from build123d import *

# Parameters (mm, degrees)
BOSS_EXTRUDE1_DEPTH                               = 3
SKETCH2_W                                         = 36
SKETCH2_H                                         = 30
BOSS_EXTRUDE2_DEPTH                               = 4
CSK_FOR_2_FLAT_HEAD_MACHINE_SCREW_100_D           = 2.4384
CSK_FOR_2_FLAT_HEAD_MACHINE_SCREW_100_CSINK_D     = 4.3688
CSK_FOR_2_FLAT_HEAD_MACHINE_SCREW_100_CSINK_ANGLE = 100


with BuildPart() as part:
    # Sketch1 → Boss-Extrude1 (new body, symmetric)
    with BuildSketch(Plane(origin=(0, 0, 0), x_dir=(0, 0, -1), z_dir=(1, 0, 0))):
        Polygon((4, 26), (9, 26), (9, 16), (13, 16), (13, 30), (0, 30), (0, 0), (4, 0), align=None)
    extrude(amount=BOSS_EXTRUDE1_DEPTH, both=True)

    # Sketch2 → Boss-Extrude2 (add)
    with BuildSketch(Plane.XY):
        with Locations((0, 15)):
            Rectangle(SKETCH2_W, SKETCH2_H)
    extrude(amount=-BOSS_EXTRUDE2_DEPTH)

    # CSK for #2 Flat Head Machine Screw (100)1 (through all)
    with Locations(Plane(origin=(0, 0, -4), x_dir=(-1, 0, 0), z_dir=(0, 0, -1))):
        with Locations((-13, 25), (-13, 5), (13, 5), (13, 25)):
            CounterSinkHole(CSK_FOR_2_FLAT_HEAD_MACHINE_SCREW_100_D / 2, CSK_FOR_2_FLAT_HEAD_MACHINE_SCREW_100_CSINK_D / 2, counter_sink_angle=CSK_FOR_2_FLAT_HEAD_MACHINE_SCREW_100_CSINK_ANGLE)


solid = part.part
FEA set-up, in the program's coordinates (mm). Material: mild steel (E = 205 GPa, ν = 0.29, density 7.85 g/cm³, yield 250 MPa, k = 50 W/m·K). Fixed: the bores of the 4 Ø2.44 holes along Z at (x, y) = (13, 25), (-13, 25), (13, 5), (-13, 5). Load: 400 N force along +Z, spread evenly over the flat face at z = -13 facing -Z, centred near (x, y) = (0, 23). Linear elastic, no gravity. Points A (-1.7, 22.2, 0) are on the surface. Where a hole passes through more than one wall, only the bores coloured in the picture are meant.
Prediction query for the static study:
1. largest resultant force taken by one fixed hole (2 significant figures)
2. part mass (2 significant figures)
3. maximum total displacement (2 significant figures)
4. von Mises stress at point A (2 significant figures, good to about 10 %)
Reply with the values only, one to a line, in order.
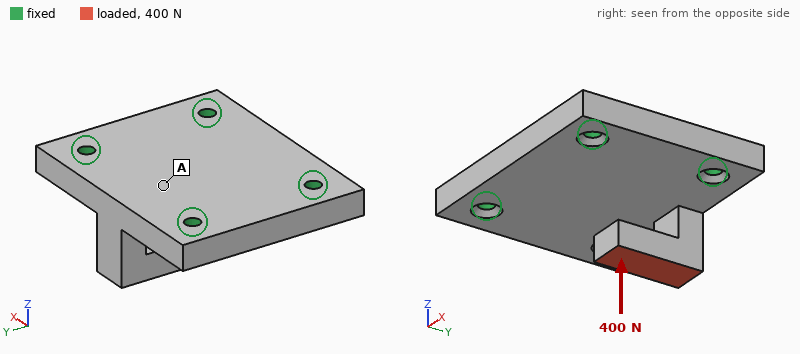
190 N
37 g
46 µm
23 MPa
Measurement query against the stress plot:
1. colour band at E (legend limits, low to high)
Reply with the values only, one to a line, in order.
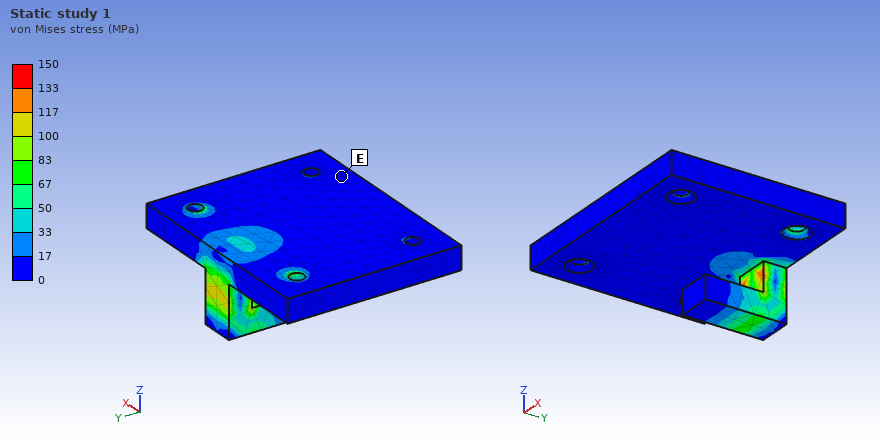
0 to 17 MPa
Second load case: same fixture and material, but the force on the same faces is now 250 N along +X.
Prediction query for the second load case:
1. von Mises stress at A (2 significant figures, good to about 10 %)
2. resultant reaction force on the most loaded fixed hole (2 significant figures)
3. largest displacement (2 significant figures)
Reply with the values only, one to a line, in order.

13 MPa
180 N
32 µm
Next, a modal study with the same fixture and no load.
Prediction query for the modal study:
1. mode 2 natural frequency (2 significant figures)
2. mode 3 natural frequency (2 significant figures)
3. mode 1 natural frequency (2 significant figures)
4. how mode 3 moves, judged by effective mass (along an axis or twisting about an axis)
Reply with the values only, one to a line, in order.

11 kHz
17 kHz
9100 Hz
along Z
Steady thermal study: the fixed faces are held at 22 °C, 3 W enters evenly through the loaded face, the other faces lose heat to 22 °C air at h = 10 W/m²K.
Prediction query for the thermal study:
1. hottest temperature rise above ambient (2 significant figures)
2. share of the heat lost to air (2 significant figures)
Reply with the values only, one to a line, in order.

37 K
4.1 %
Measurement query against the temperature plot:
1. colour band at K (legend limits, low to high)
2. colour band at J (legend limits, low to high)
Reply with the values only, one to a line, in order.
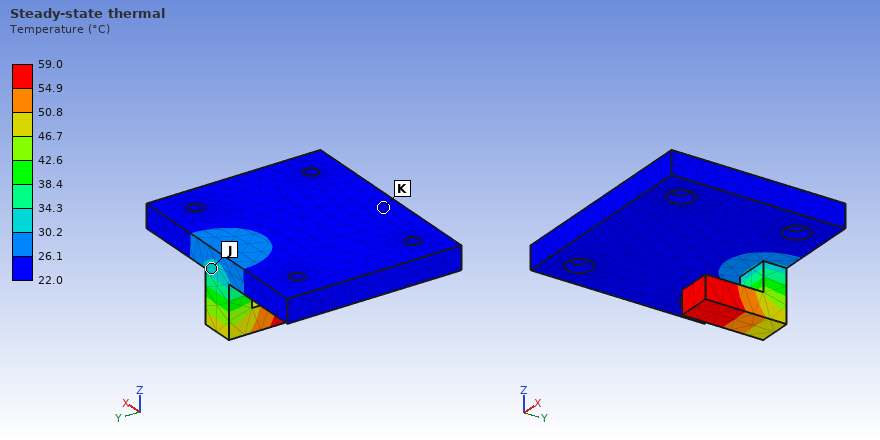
22.0 to 26.1 °C
30.2 to 34.3 °C
